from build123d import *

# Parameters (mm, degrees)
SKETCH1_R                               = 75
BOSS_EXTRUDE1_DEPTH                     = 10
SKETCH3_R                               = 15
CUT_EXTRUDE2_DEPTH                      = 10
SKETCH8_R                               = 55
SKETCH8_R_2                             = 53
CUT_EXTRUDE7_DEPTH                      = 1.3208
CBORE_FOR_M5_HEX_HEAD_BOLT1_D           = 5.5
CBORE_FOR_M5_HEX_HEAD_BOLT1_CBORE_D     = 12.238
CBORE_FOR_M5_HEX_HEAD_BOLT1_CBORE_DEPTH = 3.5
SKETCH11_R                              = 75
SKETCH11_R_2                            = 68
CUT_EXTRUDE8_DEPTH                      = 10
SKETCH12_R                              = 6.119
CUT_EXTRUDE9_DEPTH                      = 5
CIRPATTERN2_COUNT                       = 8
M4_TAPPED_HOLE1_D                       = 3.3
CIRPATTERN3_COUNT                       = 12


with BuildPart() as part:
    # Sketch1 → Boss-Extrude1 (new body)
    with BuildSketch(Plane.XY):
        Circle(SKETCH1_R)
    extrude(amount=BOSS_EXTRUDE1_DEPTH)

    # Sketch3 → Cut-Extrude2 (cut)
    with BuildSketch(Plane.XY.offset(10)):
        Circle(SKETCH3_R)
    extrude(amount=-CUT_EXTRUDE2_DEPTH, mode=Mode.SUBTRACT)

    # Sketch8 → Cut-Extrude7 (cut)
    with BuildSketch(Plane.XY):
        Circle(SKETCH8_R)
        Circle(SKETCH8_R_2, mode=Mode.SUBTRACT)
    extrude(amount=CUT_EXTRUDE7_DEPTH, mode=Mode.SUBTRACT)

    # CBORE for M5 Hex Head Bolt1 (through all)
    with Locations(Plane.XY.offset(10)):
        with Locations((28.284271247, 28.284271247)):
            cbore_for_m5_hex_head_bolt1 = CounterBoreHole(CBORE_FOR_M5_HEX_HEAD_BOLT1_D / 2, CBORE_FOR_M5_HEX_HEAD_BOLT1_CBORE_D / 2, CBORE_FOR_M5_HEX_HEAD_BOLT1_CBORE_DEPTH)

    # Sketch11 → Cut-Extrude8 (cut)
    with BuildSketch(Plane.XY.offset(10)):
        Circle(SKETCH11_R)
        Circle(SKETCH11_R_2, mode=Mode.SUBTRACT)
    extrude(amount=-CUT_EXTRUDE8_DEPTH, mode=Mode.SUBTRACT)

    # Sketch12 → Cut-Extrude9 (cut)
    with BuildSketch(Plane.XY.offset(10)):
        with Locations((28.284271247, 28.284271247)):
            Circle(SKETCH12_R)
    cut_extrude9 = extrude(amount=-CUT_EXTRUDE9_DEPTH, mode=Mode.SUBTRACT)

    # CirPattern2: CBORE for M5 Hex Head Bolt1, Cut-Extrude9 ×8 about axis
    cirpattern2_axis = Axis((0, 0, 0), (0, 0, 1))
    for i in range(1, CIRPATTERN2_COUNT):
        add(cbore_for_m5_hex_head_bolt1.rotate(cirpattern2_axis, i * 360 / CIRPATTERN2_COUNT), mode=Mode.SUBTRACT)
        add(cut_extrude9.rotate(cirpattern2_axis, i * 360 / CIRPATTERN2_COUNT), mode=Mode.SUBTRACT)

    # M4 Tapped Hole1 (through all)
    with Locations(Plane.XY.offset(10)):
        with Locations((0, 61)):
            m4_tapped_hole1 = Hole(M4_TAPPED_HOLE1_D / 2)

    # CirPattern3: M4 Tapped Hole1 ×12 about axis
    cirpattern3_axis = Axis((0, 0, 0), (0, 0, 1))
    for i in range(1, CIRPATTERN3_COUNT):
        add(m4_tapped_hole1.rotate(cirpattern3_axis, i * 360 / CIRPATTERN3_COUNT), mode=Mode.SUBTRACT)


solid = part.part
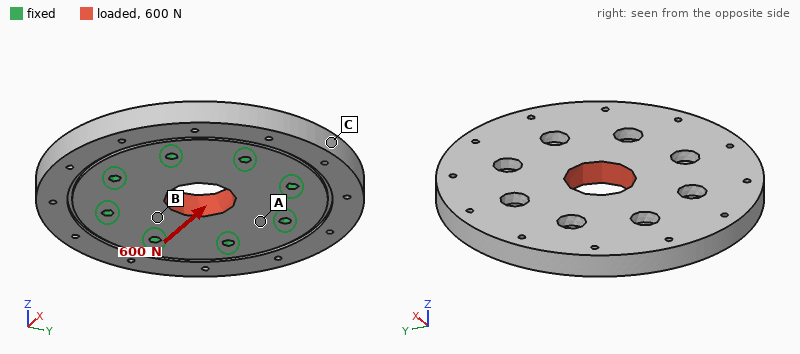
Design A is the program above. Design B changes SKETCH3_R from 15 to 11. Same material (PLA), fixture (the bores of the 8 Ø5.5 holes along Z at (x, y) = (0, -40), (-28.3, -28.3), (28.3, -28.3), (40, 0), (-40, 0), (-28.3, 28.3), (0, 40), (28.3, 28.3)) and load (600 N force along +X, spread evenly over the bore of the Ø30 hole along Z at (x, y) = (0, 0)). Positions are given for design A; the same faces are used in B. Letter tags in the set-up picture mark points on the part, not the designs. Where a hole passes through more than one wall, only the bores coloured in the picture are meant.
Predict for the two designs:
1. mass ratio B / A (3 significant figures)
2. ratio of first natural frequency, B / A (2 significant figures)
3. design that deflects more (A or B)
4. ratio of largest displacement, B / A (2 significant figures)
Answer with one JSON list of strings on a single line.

["1.03", "1.0", "B", "1.1"]
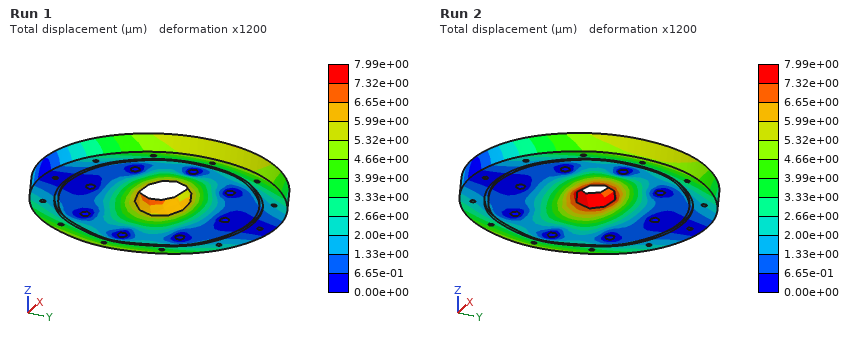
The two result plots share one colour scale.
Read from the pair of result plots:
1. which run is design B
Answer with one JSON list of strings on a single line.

["Run 2"]
